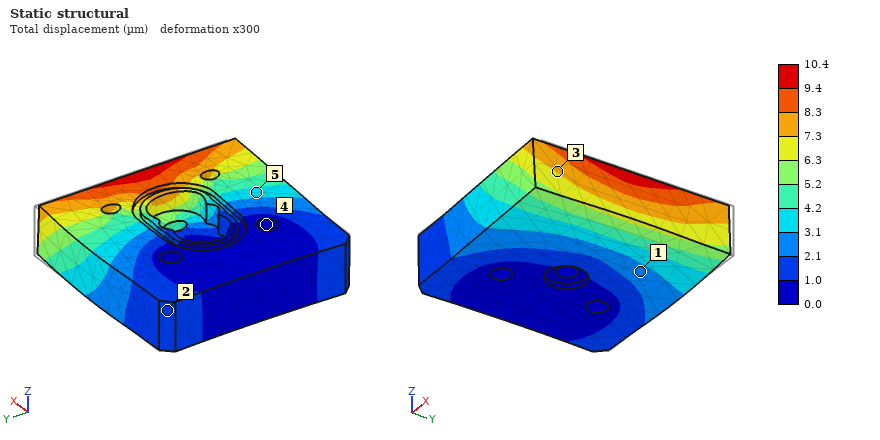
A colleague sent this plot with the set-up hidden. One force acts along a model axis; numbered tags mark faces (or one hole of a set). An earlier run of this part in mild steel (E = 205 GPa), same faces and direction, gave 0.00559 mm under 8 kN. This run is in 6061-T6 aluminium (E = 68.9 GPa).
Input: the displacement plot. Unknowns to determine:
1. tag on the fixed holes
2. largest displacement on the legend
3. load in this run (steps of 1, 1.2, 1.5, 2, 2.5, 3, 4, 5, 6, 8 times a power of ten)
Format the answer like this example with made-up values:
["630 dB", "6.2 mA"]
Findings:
["4", "10.4 µm", "5 kN"]
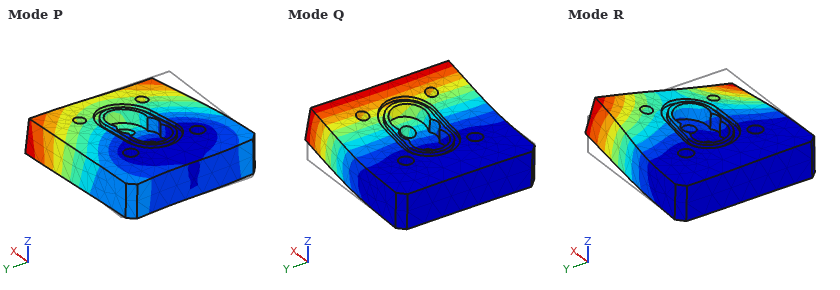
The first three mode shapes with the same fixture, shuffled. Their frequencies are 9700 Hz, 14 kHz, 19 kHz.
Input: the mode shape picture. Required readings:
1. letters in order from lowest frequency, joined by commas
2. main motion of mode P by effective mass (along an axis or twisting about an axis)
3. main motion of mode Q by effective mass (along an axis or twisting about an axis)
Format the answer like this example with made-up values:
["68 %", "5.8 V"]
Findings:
["Q, R, P", "along Y", "along Z"]
